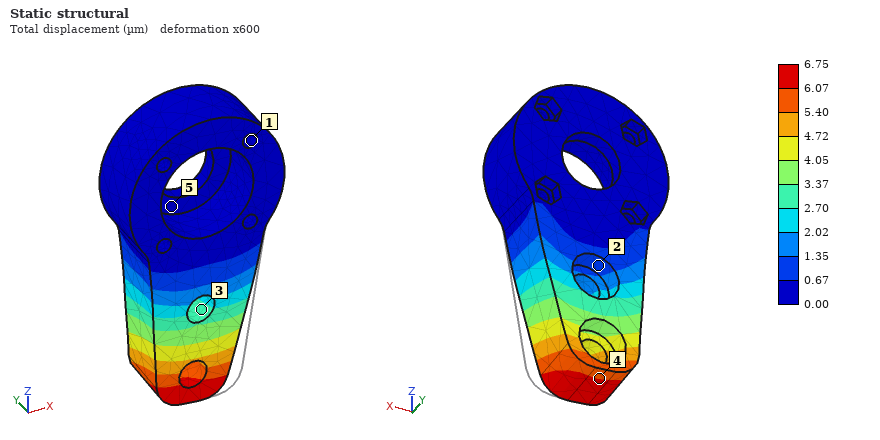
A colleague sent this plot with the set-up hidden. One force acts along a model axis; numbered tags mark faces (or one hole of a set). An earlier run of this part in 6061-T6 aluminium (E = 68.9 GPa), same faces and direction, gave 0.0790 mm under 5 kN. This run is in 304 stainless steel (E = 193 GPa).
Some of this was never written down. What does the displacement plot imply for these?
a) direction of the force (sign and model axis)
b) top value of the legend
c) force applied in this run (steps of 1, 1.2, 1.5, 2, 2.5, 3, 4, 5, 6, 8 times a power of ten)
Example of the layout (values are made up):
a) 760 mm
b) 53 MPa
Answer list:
a) -X
b) 6.75 µm
c) 1.2 kN
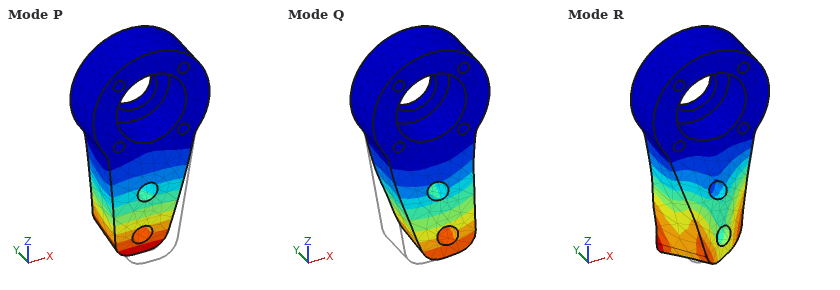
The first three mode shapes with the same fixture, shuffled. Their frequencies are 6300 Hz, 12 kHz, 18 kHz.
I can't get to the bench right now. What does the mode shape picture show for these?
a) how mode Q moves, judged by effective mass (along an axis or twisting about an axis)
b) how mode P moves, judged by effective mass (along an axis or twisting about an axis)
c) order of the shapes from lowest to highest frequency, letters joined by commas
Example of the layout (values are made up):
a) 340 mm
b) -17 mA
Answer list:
a) along X
b) along Y
c) P, Q, R
